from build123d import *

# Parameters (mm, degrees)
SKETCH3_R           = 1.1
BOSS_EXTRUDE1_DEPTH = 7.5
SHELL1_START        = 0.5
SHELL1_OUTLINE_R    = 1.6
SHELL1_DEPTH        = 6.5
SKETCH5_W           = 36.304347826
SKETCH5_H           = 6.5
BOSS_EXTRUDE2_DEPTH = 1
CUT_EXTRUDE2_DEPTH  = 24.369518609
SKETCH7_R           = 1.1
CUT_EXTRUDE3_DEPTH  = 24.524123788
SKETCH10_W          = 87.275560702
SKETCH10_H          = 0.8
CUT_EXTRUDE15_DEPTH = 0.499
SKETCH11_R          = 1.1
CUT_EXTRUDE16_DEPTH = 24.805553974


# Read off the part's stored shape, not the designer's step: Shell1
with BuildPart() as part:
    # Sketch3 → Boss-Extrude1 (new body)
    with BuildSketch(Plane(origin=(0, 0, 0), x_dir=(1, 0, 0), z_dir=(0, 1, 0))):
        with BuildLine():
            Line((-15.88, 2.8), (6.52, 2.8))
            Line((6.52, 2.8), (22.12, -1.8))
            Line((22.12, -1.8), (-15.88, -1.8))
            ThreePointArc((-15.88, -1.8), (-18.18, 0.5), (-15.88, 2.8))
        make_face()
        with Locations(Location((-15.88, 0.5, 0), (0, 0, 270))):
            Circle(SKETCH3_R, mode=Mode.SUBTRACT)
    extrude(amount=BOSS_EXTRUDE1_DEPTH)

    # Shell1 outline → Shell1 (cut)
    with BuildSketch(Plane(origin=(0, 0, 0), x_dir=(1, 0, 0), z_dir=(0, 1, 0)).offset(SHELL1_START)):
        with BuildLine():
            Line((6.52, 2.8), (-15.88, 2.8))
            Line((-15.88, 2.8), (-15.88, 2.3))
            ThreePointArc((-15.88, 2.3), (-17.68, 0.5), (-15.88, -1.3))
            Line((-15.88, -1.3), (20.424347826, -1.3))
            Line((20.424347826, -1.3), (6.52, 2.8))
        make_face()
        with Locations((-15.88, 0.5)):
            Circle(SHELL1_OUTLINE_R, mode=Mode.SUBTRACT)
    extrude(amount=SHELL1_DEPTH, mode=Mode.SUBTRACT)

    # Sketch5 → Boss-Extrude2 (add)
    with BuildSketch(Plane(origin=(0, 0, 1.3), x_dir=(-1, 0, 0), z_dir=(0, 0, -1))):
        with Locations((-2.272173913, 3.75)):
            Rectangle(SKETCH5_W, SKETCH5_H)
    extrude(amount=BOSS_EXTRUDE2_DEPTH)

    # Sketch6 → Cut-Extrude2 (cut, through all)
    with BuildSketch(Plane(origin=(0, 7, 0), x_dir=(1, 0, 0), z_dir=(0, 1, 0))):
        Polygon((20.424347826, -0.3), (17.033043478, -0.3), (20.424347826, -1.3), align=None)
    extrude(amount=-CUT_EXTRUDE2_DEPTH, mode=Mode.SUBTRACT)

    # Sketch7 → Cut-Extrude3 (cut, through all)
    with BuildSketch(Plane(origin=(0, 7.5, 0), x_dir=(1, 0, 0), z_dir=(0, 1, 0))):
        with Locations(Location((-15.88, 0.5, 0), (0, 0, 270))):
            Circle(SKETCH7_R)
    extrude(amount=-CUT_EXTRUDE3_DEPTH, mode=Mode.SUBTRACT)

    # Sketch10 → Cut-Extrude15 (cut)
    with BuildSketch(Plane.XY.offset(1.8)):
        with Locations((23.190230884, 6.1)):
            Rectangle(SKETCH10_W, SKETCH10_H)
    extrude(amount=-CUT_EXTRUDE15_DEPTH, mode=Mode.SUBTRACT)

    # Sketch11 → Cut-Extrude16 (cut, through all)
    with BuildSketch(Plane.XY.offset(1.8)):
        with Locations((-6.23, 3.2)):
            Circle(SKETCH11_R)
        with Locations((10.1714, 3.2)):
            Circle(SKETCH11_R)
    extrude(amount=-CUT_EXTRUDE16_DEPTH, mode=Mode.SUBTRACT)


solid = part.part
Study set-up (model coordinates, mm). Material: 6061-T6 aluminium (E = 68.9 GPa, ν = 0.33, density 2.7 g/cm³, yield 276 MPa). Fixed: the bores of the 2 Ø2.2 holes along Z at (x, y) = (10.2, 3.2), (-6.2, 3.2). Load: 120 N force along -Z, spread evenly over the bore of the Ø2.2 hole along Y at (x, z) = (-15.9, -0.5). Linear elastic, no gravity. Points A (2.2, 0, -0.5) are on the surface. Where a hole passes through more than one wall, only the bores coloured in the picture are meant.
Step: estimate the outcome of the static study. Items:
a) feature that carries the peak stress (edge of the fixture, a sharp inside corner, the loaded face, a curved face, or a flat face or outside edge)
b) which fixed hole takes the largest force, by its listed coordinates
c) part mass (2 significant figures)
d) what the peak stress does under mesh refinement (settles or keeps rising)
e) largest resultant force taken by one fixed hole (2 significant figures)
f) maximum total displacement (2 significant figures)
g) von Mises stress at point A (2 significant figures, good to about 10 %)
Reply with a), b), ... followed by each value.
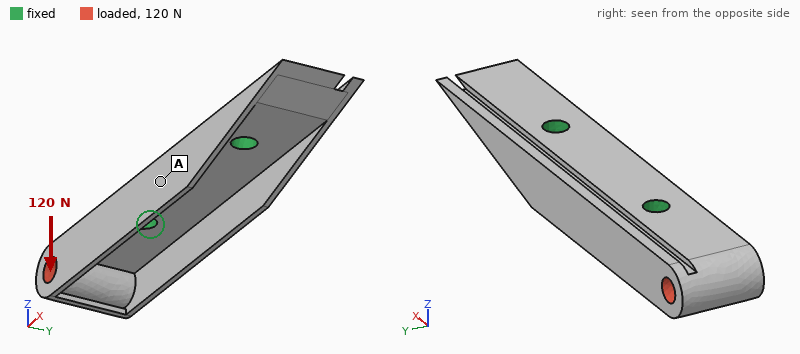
a) edge of the fixture
b) (-6.2, 3.2)
c) 1.4 g
d) keeps rising
e) 180 N
f) 86 µm
g) 28 MPa
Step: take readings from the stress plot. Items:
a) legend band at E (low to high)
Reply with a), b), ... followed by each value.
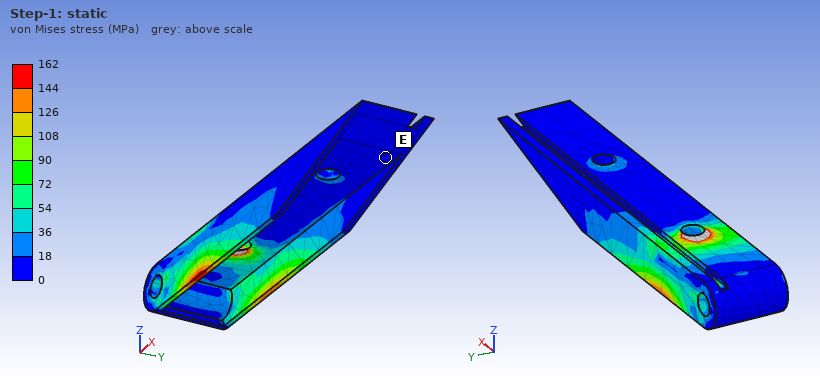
a) 0 to 18 MPa
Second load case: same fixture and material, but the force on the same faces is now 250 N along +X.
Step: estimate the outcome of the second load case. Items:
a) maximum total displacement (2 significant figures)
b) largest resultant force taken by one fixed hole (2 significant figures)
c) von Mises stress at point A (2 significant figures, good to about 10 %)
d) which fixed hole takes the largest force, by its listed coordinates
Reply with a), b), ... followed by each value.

a) 29 µm
b) 200 N
c) 11 MPa
d) (-6.2, 3.2)
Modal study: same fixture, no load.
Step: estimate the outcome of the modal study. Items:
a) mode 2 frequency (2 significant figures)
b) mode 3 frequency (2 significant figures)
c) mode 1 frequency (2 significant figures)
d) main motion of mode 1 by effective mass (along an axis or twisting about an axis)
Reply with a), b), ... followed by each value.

a) 18 kHz
b) 18 kHz
c) 13 kHz
d) along Z
